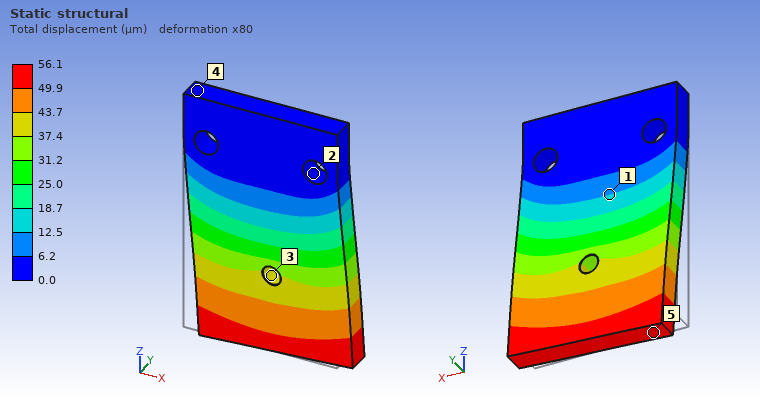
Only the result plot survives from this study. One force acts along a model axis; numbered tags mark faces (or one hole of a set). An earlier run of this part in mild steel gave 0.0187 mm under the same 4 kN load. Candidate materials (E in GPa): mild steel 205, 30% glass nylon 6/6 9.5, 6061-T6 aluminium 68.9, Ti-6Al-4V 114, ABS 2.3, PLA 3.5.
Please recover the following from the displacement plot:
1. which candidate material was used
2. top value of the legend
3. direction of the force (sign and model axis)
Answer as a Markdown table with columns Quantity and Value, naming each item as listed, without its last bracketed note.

| Quantity | Value |
|---|---|
| which candidate material was used | 6061-T6 aluminium |
| top value of the legend | 56.1 µm |
| direction of the force | +X |
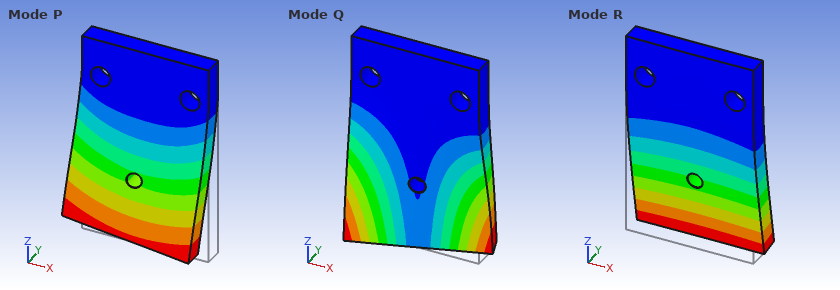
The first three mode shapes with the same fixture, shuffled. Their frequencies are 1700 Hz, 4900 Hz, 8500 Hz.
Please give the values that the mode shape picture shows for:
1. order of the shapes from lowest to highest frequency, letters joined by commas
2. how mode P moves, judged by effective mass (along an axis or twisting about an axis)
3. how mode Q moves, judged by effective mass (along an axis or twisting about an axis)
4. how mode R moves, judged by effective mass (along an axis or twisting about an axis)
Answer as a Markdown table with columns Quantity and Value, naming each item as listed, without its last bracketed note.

| Quantity | Value |
|---|---|
| order of the shapes from lowest to highest frequency, letters joined by commas | R, Q, P |
| how mode P moves, judged by effective mass | along X |
| how mode Q moves, judged by effective mass | twisting about Z |
| how mode R moves, judged by effective mass | along Y |
